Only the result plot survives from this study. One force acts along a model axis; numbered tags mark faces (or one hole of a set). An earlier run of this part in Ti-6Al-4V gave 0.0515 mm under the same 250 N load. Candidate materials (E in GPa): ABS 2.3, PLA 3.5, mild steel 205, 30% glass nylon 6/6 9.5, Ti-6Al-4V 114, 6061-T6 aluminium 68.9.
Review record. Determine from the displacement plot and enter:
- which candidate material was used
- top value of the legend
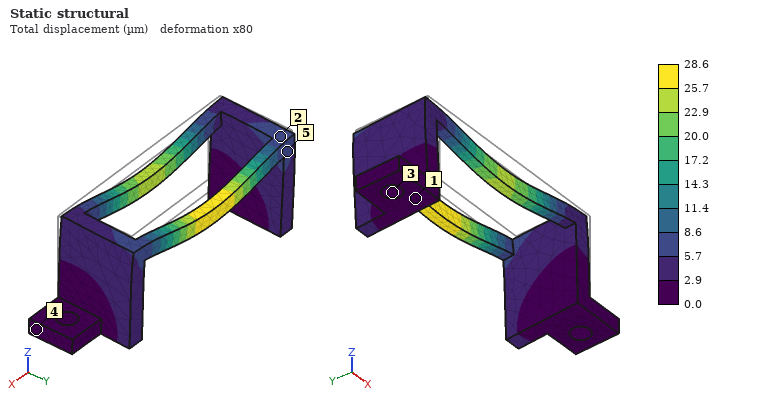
mild steel
28.6 µm
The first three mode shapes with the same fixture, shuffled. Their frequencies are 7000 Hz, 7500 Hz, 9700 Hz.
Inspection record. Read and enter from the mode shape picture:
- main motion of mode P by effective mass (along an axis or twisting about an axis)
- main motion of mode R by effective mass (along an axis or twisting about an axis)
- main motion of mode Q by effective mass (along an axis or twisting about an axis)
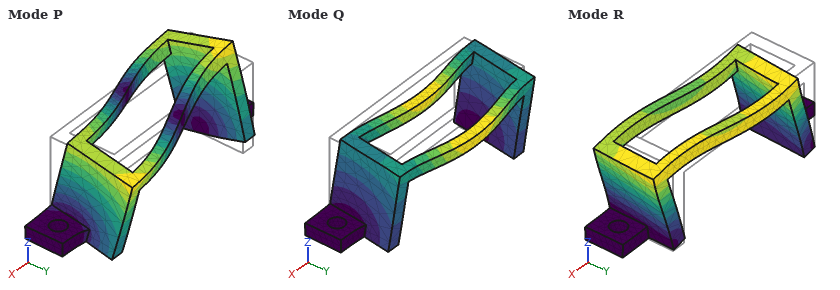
twisting about Z
along X
along Y
